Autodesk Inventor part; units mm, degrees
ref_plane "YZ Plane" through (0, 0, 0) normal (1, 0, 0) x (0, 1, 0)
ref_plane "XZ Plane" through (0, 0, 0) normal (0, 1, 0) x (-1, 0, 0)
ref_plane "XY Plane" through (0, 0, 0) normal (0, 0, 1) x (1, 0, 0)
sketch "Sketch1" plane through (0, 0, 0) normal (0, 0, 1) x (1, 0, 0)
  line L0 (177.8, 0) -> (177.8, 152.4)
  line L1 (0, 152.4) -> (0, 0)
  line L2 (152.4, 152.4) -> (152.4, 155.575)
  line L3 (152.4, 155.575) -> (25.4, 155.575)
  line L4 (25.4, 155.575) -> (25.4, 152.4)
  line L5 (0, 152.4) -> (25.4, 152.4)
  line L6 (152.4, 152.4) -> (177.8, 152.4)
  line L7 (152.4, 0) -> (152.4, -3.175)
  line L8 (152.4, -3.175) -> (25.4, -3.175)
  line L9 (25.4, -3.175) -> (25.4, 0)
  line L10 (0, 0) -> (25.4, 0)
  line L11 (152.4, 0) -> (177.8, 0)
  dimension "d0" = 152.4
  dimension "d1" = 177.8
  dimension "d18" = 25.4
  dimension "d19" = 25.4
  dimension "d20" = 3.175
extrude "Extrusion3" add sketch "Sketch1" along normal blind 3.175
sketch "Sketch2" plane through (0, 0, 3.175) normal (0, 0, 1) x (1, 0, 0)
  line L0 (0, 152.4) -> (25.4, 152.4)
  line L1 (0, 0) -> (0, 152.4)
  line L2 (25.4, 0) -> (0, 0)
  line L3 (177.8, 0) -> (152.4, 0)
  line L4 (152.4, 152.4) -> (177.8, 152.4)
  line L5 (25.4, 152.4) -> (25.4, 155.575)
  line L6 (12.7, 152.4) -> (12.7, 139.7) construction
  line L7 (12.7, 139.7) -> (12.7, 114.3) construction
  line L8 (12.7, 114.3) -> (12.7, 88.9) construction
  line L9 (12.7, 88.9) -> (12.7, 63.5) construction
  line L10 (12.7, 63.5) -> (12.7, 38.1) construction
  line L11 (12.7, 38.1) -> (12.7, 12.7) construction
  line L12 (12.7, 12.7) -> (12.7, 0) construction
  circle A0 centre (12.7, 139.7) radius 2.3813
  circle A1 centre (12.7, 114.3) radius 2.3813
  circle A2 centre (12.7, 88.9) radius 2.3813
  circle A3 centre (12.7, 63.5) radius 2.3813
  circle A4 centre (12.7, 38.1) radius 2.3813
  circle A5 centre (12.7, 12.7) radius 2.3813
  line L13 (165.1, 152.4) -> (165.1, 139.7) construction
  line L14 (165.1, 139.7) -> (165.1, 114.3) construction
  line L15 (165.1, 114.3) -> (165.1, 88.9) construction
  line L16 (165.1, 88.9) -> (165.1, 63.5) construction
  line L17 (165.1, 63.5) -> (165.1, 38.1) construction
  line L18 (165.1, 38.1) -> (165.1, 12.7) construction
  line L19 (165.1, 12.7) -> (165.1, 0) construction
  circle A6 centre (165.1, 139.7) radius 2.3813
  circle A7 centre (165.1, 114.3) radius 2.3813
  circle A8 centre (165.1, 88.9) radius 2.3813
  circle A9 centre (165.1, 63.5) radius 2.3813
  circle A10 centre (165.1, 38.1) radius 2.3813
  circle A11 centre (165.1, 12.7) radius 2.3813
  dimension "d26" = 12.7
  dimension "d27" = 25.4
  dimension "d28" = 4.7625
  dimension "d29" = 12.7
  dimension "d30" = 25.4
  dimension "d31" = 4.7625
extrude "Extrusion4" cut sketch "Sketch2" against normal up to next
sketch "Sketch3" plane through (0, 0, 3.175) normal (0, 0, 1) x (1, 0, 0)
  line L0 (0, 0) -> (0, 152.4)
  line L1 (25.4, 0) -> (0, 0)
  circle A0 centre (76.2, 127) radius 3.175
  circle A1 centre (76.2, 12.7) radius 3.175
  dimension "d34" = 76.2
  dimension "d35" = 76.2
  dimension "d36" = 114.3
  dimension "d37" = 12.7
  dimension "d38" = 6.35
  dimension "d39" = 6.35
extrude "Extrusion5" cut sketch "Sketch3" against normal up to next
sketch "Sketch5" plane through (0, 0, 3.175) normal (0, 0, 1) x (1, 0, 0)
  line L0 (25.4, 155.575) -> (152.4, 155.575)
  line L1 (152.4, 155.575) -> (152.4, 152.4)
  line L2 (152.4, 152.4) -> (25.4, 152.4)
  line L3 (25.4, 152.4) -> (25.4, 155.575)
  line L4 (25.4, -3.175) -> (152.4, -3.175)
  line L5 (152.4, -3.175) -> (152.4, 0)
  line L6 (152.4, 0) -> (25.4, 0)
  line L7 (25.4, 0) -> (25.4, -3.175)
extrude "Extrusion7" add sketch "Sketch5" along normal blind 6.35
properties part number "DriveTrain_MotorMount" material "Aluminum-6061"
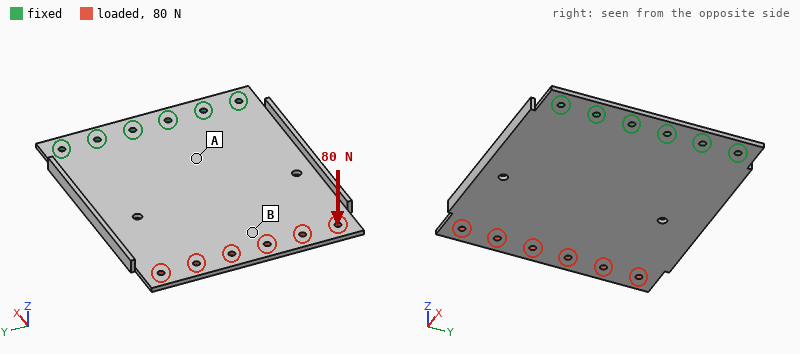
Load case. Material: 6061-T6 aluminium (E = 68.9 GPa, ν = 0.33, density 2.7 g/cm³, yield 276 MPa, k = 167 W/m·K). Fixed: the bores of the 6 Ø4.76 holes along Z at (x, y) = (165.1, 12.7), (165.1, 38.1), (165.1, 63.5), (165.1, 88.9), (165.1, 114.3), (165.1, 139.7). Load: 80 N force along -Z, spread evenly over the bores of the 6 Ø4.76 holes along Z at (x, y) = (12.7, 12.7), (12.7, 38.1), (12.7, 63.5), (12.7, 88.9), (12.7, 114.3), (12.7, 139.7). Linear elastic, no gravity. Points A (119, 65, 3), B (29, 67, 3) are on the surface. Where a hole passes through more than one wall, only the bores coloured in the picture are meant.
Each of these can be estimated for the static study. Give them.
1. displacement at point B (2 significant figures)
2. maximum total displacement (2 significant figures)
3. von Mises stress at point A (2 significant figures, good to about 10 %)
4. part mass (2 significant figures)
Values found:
1.7 mm
2.3 mm
17 MPa
250 g
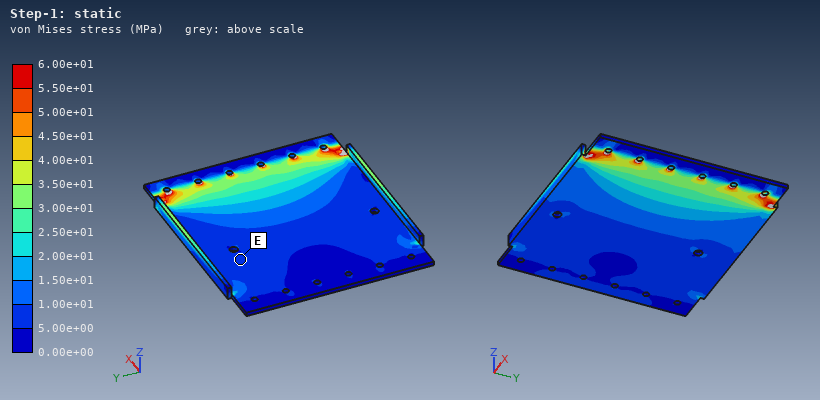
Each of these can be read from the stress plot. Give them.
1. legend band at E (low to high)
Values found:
5.00e+00 to 1.00e+01 MPa
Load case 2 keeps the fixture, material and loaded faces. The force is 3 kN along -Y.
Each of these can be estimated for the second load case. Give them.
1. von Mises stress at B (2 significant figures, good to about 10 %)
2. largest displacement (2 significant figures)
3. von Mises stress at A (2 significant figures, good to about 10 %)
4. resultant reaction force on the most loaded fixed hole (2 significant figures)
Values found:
17 MPa
0.14 mm
16 MPa
2.9 kN
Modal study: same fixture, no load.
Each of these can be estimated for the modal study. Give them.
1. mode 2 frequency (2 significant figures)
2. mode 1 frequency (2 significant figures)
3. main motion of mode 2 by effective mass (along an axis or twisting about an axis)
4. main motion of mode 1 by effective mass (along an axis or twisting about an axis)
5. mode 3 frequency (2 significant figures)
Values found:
250 Hz
120 Hz
twisting about X
along Z
730 Hz
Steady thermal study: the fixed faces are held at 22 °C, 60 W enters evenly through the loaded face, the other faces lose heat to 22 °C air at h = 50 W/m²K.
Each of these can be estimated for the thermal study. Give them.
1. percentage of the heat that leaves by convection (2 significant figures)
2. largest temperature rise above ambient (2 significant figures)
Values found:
81 %
45 K
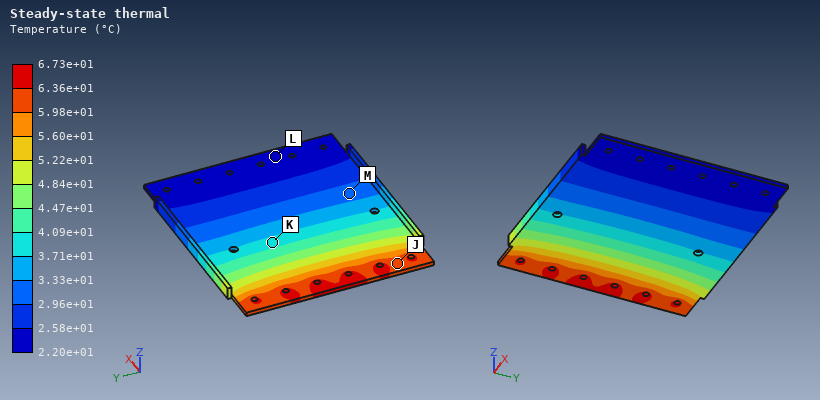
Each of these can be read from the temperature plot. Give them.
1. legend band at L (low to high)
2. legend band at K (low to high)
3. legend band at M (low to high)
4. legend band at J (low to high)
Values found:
2.20e+01 to 2.58e+01 °C
3.71e+01 to 4.09e+01 °C
2.96e+01 to 3.33e+01 °C
5.98e+01 to 6.36e+01 °C
